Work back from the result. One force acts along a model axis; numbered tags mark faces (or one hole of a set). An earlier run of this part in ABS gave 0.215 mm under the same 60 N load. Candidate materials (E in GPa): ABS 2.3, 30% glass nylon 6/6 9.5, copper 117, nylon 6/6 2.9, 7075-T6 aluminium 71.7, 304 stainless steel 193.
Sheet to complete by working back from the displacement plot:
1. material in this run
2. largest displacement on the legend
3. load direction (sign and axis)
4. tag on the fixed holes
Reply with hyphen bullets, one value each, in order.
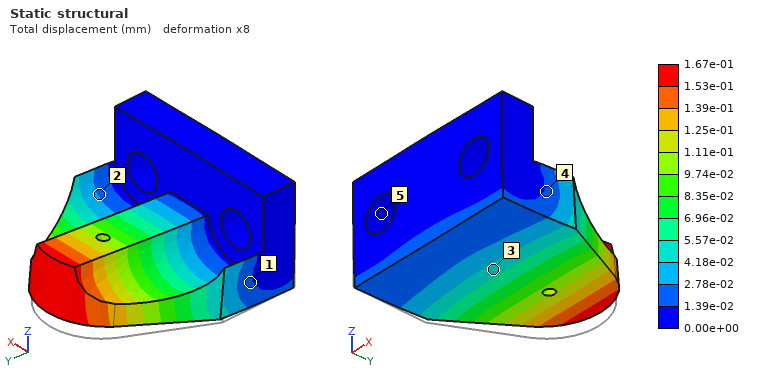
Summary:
- nylon 6/6
- 1.67e-01 mm
- +Z
- 5
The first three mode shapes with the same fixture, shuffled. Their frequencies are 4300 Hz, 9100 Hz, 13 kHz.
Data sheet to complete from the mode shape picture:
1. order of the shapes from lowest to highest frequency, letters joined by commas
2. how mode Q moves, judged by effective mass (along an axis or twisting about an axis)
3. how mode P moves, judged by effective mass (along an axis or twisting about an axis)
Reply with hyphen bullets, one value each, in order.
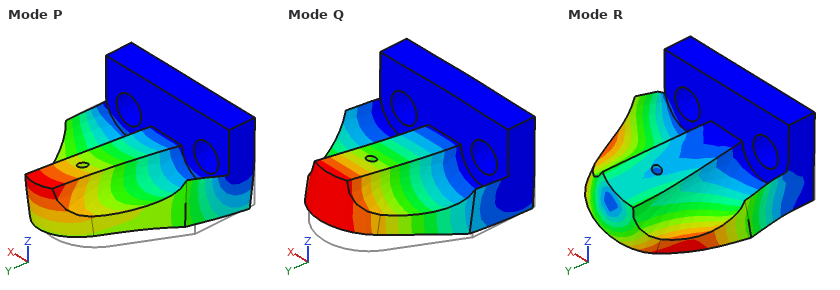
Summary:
- Q, P, R
- along Z
- along X
